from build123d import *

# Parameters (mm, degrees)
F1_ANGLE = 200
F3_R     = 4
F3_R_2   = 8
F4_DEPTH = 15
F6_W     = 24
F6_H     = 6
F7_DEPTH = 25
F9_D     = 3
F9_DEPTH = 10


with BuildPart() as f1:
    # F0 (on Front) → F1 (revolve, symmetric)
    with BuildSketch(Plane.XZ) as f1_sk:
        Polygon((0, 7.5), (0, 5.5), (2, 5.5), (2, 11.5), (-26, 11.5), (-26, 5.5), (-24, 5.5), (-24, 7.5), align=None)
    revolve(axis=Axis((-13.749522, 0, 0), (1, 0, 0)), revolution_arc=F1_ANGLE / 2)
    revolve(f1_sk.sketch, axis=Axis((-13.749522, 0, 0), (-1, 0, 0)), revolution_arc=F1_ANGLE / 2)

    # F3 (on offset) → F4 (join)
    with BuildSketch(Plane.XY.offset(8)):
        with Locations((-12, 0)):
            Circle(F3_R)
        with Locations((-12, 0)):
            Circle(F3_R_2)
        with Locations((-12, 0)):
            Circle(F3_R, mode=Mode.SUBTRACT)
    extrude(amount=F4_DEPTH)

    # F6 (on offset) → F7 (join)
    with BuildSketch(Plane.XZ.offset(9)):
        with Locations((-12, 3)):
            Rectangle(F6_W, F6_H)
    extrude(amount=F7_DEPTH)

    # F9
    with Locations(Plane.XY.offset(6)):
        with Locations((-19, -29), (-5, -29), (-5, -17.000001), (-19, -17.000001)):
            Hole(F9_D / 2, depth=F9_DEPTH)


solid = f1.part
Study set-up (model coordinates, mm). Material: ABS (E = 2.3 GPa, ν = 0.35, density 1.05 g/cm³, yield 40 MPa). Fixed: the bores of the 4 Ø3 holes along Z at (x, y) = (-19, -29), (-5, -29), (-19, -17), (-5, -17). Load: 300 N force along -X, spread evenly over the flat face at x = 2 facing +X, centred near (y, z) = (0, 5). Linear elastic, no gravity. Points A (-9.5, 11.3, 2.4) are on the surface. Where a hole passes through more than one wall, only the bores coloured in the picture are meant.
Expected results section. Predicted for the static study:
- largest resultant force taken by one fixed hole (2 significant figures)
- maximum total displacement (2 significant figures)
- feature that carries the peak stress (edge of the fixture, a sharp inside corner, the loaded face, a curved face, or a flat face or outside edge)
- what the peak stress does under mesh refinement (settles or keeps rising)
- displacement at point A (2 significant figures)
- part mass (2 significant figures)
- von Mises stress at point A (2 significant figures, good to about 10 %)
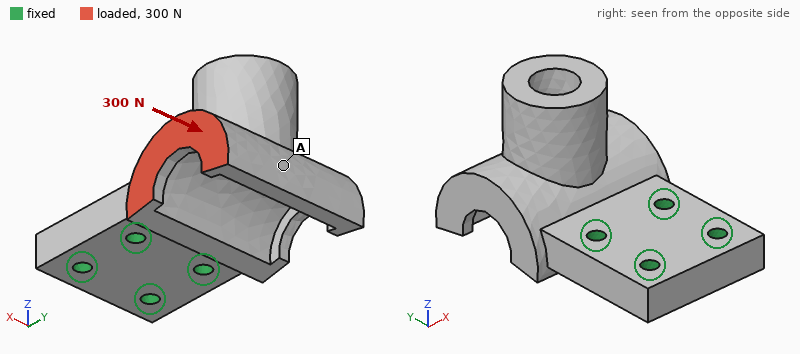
310 N
0.37 mm
edge of the fixture
keeps rising
0.28 mm
9.4 g
1.6 MPa
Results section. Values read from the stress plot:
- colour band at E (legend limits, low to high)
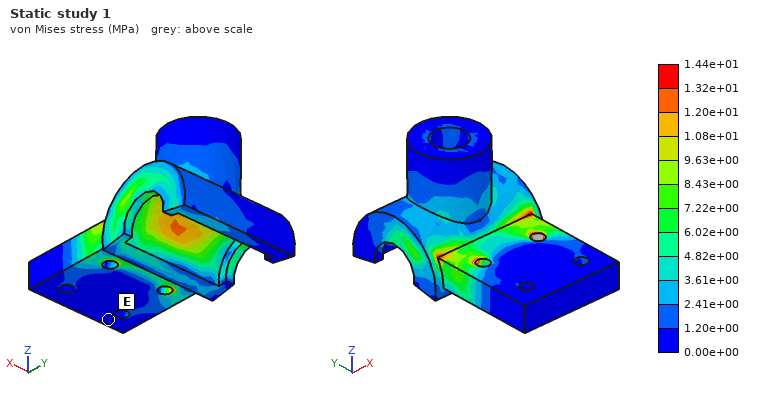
0.00e+00 to 1.20e+00 MPa
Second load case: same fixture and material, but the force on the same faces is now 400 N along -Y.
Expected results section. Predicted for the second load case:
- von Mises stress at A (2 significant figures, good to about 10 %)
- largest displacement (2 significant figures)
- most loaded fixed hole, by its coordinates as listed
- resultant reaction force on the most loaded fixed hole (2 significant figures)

6.4 MPa
0.54 mm
(-5, -17)
480 N
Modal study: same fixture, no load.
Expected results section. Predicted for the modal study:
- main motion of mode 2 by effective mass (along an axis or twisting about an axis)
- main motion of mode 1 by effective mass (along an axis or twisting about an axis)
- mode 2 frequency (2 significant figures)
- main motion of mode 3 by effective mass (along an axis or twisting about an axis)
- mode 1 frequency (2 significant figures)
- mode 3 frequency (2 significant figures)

twisting about Y
along Z
2300 Hz
along X
990 Hz
2900 Hz
